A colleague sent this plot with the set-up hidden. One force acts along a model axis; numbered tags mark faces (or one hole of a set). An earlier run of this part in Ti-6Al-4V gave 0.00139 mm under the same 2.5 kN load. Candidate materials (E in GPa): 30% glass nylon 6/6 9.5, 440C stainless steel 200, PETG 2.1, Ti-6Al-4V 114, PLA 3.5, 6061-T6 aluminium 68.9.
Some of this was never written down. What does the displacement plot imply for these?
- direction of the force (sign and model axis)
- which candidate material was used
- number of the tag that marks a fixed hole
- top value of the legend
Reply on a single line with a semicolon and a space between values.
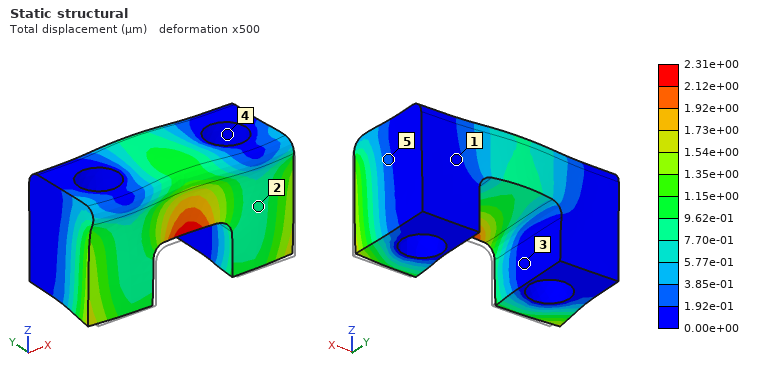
+Y; 6061-T6 aluminium; 4; 2.31e+00 µm
